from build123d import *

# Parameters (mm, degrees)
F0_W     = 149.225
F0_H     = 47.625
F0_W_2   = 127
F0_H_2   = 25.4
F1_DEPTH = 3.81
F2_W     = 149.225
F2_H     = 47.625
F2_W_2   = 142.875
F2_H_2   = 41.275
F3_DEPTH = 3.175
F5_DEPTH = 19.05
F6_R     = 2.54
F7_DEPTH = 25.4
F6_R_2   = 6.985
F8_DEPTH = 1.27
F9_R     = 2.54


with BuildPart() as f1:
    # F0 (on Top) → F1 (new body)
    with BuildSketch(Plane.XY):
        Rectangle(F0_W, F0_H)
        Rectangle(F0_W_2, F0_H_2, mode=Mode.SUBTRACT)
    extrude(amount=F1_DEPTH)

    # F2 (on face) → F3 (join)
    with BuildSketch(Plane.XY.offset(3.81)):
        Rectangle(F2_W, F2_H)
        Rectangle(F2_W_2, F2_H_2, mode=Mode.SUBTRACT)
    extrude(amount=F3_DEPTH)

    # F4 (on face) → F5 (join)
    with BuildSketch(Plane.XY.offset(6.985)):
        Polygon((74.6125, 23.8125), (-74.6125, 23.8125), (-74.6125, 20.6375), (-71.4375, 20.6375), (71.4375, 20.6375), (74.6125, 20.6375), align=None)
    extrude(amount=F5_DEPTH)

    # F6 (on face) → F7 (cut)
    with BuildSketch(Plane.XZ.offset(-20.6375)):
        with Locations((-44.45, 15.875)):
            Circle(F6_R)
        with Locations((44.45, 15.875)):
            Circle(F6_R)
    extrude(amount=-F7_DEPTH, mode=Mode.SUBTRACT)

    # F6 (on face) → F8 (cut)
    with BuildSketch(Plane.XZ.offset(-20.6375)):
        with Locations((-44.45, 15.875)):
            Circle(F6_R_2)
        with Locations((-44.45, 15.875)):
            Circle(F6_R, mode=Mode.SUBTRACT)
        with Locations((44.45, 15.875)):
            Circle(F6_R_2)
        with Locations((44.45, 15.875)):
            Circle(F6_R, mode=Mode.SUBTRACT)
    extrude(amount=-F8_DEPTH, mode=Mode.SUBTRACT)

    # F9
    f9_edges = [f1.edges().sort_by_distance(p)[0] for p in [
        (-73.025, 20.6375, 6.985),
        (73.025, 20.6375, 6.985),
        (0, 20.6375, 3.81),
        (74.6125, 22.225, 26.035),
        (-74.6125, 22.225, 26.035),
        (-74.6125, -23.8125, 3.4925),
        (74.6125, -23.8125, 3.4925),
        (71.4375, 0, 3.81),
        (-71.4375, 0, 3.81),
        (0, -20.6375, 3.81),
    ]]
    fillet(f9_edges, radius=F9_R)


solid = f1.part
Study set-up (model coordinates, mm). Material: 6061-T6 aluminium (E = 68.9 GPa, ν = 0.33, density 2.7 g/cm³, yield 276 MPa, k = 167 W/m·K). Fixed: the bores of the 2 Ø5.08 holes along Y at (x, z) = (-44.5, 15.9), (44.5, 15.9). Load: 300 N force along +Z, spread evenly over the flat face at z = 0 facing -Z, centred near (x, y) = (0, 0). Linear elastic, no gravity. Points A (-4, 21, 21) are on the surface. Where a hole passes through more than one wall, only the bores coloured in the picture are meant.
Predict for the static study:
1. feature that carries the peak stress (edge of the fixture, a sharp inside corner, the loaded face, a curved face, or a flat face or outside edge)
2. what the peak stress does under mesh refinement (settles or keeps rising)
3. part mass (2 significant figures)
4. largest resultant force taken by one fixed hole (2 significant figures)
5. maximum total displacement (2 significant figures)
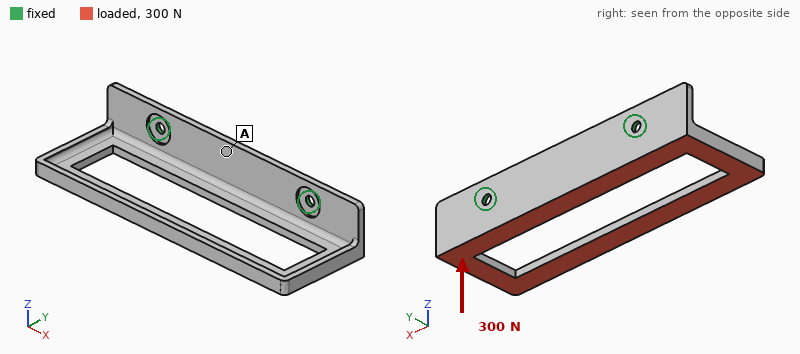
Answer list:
edge of the fixture
keeps rising
75 g
170 N
0.97 mm
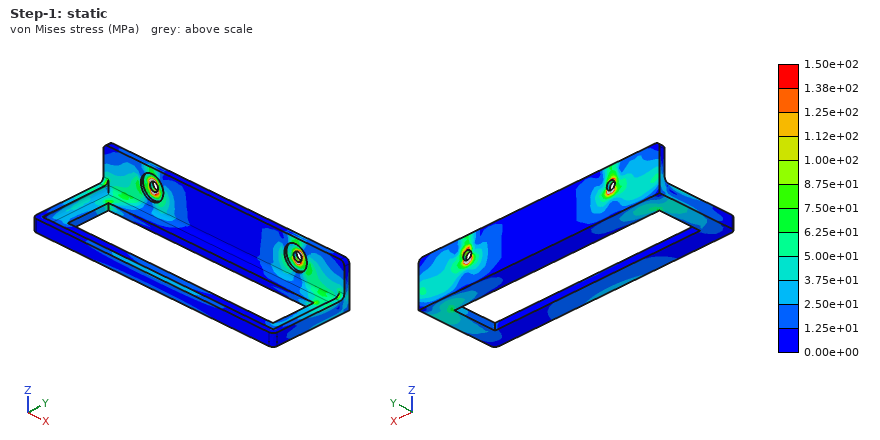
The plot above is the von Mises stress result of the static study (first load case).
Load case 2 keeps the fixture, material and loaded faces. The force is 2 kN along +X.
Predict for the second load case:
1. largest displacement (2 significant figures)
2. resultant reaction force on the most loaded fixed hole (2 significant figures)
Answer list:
0.69 mm
1.2 kN
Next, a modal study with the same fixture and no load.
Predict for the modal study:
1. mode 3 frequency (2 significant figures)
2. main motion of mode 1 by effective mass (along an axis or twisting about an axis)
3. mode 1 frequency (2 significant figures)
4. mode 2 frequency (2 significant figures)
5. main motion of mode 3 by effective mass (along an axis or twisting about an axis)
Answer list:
1300 Hz
along Z
440 Hz
850 Hz
along Y
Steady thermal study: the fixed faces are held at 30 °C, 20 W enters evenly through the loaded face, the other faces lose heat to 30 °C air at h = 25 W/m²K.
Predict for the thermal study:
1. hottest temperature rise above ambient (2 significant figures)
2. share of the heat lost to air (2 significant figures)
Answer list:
35 K
25 %
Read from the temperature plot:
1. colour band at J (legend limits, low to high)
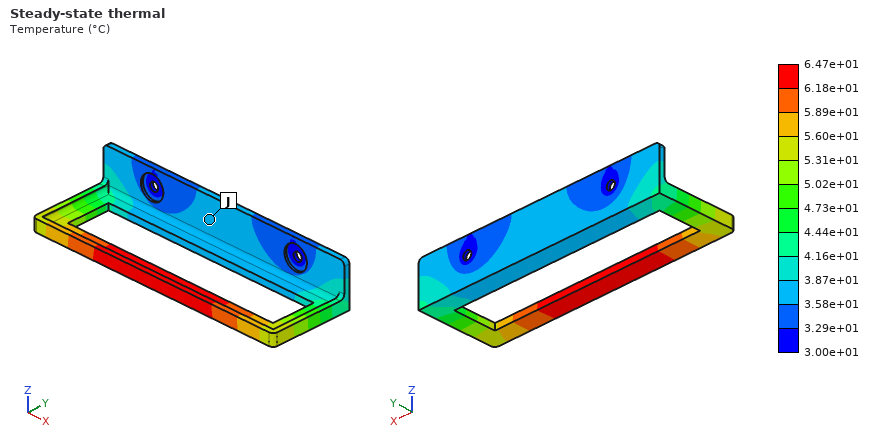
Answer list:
3.58e+01 to 3.87e+01 °C
